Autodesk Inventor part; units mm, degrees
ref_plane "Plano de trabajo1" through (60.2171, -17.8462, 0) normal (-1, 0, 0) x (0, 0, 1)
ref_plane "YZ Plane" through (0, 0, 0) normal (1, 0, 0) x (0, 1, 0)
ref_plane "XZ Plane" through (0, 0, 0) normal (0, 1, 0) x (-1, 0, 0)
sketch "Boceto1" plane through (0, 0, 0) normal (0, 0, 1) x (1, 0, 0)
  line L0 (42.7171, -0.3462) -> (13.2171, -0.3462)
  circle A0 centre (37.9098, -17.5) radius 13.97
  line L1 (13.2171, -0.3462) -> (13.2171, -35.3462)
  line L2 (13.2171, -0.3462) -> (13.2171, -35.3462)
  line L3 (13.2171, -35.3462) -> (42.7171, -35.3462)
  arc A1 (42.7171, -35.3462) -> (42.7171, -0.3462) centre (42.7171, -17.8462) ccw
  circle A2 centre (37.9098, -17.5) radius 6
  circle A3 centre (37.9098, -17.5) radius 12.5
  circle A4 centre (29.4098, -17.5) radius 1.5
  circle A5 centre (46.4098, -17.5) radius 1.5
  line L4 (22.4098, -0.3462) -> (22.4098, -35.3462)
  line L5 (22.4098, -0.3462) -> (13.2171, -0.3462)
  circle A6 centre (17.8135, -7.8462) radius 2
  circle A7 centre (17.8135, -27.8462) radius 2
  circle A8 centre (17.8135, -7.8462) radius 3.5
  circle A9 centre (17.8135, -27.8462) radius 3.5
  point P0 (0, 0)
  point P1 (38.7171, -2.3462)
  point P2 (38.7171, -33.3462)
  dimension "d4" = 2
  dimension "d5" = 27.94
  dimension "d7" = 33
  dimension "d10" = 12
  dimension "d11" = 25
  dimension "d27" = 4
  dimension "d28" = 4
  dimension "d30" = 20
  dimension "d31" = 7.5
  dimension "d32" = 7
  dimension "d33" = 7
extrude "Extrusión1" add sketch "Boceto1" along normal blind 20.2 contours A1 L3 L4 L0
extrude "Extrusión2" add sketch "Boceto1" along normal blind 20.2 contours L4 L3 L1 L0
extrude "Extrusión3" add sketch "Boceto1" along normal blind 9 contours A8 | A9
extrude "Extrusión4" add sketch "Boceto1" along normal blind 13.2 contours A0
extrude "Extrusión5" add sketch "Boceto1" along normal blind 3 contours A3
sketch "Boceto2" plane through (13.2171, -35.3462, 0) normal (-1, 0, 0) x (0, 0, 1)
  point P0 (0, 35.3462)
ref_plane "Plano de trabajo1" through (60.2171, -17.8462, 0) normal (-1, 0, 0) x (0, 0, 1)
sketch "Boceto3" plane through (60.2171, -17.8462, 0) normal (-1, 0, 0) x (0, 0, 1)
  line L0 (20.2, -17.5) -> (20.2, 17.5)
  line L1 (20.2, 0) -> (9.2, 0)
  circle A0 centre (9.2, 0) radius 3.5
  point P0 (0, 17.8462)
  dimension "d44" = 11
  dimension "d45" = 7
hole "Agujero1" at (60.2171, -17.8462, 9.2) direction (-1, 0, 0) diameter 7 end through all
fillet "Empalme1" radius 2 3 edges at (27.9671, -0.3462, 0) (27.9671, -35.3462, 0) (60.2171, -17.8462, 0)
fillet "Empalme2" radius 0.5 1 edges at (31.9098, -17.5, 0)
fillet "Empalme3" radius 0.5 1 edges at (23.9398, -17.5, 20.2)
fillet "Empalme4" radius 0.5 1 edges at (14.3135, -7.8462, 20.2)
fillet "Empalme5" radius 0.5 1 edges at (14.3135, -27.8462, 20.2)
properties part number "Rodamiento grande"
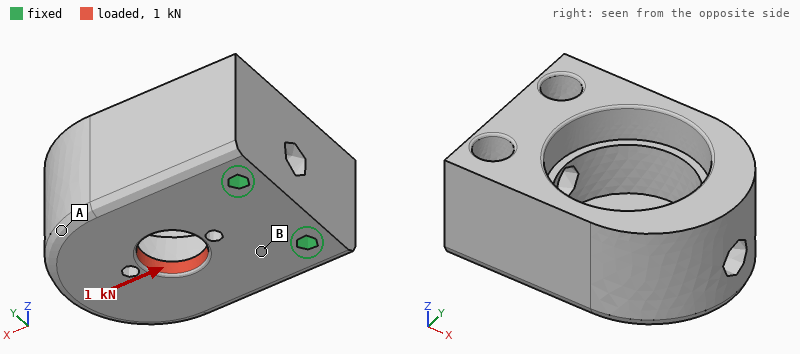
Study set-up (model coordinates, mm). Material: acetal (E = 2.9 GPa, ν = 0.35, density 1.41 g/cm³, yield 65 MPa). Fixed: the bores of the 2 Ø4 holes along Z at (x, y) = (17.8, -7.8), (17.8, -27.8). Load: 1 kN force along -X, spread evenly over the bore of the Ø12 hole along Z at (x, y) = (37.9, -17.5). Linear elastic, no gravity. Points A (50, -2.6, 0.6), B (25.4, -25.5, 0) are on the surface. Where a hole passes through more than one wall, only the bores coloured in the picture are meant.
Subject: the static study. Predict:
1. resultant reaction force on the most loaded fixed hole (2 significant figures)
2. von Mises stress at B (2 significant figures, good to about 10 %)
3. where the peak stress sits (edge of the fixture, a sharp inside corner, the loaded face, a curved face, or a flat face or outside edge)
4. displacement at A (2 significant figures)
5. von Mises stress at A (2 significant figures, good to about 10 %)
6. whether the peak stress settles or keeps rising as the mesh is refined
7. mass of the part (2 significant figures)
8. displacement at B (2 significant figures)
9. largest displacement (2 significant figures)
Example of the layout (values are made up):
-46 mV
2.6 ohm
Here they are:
520 N
11 MPa
a sharp inside corner
0.13 mm
3.1 MPa
keeps rising
27 g
0.032 mm
0.18 mm
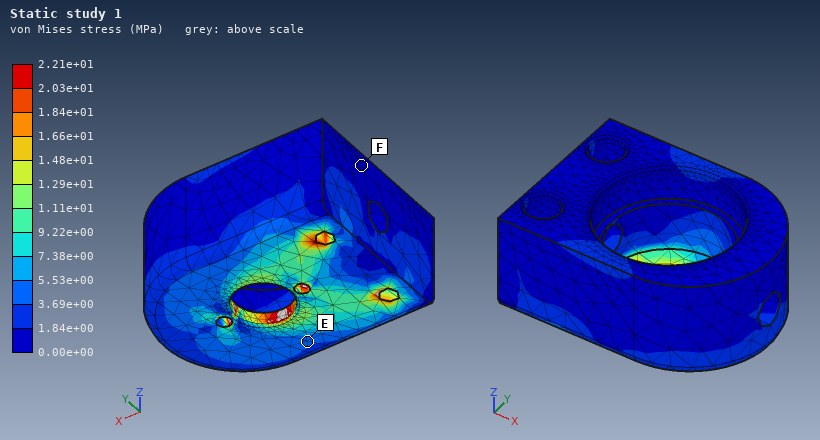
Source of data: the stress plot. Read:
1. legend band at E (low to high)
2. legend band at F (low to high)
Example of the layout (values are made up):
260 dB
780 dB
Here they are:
3.69e+00 to 5.53e+00 MPa
0.00e+00 to 1.84e+00 MPa
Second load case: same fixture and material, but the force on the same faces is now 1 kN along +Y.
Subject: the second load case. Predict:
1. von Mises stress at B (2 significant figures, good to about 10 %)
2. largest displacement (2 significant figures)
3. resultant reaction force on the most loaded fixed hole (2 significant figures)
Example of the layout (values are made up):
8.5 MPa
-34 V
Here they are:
12 MPa
0.33 mm
950 N
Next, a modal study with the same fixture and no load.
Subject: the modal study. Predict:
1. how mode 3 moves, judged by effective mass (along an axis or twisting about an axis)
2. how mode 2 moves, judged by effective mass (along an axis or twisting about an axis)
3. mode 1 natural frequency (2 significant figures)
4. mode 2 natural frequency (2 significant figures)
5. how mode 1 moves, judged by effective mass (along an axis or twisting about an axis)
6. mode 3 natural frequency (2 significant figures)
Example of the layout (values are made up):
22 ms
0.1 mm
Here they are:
twisting about X
along Y
1300 Hz
2000 Hz
along Z
3200 Hz
